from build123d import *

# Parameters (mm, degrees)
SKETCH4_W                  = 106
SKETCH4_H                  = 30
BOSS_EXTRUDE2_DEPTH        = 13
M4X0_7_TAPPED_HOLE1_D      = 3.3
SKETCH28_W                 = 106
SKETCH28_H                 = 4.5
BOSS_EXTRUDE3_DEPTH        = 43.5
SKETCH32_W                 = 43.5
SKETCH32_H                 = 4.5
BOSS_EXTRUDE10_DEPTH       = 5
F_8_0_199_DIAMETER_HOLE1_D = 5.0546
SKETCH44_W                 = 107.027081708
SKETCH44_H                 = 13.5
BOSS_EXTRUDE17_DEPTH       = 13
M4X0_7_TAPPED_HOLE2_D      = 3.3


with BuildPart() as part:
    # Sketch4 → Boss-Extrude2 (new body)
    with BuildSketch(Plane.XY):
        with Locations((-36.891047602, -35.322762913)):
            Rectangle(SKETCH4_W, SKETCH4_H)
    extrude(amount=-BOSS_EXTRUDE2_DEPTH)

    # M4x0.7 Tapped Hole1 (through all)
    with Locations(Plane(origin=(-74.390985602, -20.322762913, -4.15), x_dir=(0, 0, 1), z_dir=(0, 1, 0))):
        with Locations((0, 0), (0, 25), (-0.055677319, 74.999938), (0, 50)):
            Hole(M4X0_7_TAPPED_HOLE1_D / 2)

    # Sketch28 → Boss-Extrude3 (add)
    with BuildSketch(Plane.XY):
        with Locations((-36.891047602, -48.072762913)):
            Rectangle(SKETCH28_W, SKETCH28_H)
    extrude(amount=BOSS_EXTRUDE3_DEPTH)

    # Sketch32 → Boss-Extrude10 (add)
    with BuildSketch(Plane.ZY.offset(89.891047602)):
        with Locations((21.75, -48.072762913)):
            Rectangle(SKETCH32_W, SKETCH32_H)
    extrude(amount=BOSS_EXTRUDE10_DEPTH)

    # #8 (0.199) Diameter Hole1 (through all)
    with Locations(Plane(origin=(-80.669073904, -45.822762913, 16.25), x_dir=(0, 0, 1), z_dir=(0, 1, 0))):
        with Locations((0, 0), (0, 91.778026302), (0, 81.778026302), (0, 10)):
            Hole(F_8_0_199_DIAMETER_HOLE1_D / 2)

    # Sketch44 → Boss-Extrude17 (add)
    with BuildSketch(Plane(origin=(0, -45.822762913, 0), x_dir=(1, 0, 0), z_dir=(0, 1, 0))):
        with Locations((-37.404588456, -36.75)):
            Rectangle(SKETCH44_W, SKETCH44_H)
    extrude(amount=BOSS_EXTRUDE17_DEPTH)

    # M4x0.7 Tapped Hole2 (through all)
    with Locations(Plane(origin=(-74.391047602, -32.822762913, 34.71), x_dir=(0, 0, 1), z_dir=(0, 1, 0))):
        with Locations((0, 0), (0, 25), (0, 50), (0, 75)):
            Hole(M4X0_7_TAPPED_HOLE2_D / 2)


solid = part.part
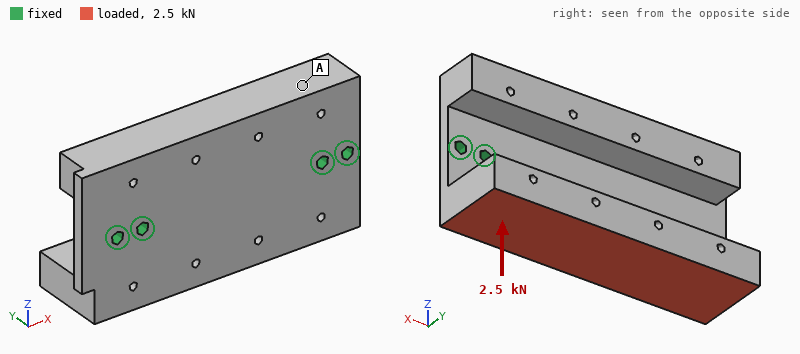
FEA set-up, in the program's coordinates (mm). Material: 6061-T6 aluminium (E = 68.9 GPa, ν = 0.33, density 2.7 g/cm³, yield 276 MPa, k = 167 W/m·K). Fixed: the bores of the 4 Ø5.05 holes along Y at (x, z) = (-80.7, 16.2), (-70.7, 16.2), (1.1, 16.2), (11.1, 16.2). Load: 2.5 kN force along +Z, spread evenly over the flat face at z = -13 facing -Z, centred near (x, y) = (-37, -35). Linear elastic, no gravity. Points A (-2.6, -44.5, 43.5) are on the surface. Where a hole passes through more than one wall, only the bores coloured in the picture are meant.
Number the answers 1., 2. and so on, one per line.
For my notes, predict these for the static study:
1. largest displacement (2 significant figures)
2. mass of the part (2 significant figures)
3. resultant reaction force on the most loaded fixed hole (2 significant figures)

1. 0.36 mm
2. 220 g
3. 1.1 kN
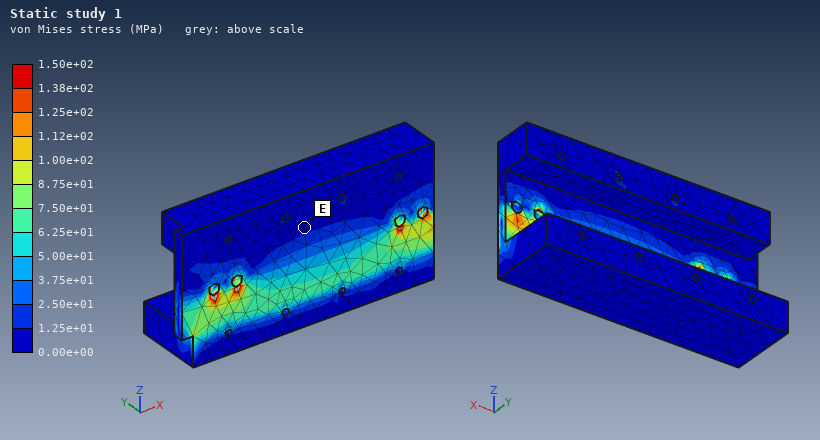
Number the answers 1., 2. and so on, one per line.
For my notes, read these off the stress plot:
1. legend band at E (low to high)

1. 0.00e+00 to 1.25e+01 MPa
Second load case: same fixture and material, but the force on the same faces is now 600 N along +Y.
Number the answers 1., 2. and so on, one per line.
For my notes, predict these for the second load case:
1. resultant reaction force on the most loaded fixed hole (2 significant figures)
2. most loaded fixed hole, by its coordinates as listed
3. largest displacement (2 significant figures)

1. 230 N
2. (1.1, 16.2)
3. 0.14 mm
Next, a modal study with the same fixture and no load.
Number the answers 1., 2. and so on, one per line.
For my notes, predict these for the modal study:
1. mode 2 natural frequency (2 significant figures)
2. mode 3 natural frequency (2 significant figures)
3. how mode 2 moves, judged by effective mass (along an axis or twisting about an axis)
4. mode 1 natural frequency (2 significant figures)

1. 2200 Hz
2. 3500 Hz
3. along Y
4. 1200 Hz
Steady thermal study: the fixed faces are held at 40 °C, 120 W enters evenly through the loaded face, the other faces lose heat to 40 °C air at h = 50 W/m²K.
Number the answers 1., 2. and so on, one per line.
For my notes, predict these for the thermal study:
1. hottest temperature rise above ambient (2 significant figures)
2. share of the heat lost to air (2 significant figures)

1. 41 K
2. 18 %
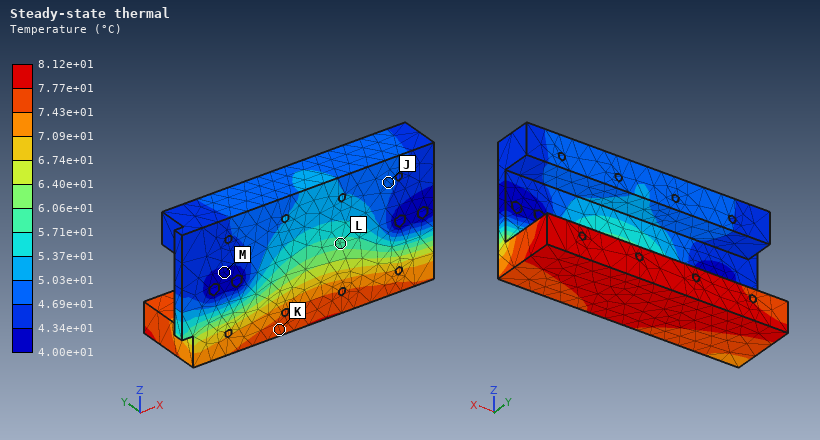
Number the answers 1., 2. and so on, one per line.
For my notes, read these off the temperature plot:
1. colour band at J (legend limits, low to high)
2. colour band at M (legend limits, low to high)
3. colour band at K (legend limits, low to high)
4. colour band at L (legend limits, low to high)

1. 4.69e+01 to 5.03e+01 °C
2. 4.00e+01 to 4.34e+01 °C
3. 7.43e+01 to 7.77e+01 °C
4. 5.71e+01 to 6.06e+01 °C
